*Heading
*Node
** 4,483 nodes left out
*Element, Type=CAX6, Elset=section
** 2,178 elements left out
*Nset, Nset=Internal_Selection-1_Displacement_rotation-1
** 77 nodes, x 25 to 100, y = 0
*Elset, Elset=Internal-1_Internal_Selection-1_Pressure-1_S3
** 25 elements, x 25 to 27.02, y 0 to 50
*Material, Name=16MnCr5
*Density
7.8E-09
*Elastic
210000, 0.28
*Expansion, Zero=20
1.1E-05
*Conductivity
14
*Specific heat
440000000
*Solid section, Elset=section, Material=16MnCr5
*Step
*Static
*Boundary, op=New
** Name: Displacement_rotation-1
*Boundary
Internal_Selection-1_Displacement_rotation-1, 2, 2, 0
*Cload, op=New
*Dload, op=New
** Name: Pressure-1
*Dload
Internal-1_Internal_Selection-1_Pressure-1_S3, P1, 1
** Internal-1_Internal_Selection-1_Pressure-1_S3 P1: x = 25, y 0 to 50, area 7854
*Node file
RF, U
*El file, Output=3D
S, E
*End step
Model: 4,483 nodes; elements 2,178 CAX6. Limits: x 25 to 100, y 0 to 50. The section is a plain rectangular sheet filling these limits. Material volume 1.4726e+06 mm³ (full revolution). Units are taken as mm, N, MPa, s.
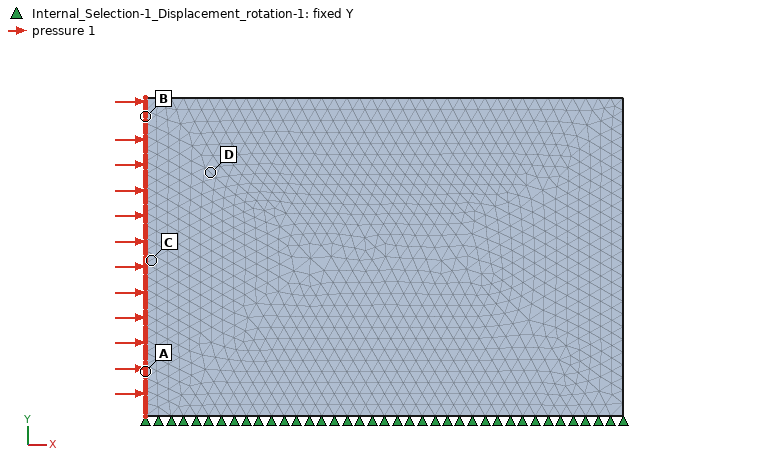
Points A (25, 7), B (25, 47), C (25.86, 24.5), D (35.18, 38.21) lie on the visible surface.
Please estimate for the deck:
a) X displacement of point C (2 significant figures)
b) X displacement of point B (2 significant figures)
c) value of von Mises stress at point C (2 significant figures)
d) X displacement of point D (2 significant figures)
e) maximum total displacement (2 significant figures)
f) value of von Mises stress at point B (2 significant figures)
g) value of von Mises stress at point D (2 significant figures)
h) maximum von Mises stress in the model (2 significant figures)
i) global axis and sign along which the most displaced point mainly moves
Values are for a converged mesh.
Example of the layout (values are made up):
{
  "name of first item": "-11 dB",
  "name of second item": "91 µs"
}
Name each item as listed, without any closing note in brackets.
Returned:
{
  "X displacement of point C": "1.6e-04 mm",
  "X displacement of point B": "1.7e-04 mm",
  "value of von Mises stress at point C": "1.7 MPa",
  "X displacement of point D": "1.2e-04 mm",
  "maximum total displacement": "1.7e-04 mm",
  "value of von Mises stress at point B": "1.8 MPa",
  "value of von Mises stress at point D": "0.93 MPa",
  "maximum von Mises stress in the model": "1.8 MPa",
  "global axis and sign along which the most displaced point mainly moves": "+X"
}
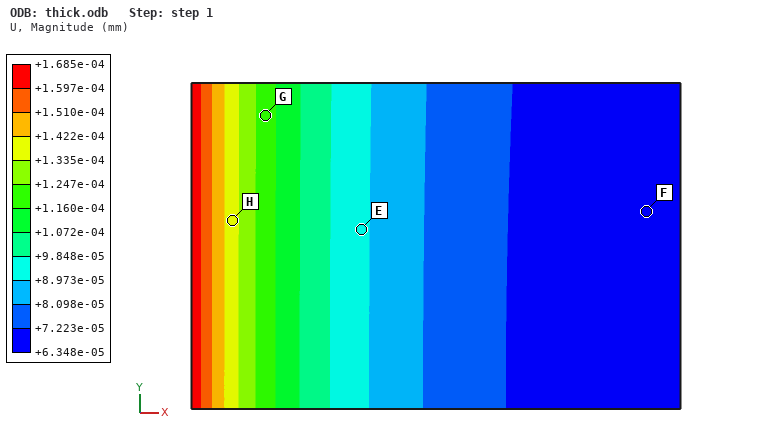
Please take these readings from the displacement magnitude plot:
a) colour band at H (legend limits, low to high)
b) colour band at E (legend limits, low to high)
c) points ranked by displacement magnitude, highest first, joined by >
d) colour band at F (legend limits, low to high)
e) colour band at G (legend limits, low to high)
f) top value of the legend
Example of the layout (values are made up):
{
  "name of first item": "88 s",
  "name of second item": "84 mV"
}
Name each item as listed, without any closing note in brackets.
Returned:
{
  "colour band at H": "+1.335e-04 to +1.422e-04 mm",
  "colour band at E": "+8.973e-05 to +9.848e-05 mm",
  "points ranked by displacement magnitude, highest first, joined by >": "H > G > E > F",
  "colour band at F": "+6.348e-05 to +7.223e-05 mm",
  "colour band at G": "+1.160e-04 to +1.247e-04 mm",
  "top value of the legend": "+1.685e-04 mm"
}
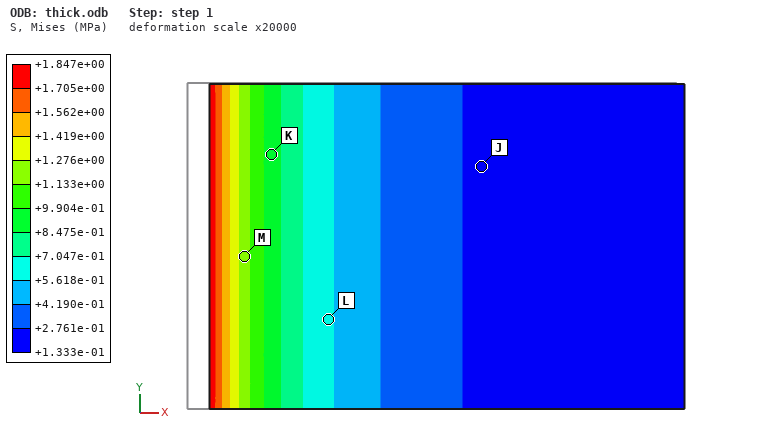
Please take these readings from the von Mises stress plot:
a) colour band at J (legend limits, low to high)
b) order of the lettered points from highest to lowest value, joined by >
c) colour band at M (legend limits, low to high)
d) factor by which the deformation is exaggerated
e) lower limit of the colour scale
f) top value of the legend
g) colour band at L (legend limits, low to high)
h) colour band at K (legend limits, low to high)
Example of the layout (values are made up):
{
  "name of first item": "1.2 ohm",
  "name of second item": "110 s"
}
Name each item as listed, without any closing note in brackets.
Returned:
{
  "colour band at J": "+1.333e-01 to +2.761e-01 MPa",
  "order of the lettered points from highest to lowest value, joined by >": "M > K > L > J",
  "colour band at M": "+1.133e+00 to +1.276e+00 MPa",
  "factor by which the deformation is exaggerated": "20000",
  "lower limit of the colour scale": "+1.333e-01 MPa",
  "top value of the legend": "+1.847e+00 MPa",
  "colour band at L": "+5.618e-01 to +7.047e-01 MPa",
  "colour band at K": "+8.475e-01 to +9.904e-01 MPa"
}
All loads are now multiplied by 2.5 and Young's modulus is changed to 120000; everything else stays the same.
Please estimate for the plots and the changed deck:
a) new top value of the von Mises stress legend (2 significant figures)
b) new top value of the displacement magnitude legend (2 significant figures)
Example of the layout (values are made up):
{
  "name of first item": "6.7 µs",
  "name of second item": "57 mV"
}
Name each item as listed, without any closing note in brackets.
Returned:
{
  "new top value of the von Mises stress legend": "4.6 MPa",
  "new top value of the displacement magnitude legend": "7.4e-04 mm"
}
